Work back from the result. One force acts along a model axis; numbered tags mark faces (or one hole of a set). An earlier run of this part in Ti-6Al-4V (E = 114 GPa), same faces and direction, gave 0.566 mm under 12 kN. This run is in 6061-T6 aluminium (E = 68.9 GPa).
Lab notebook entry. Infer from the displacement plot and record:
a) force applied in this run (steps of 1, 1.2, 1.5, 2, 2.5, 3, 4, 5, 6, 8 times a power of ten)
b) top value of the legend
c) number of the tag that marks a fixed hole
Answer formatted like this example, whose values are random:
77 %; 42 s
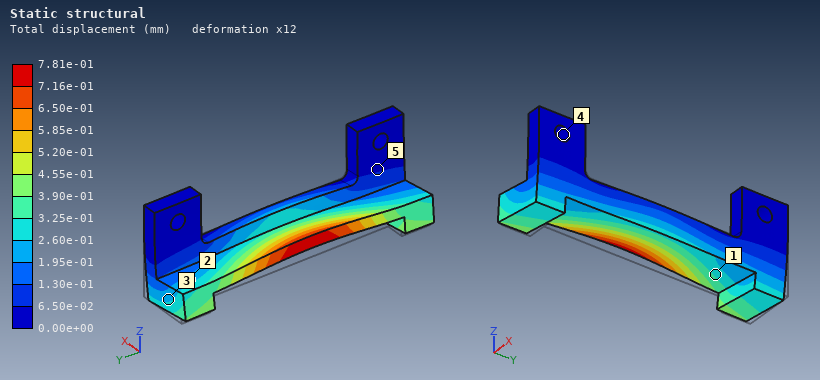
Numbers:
10 kN; 7.81e-01 mm; 4
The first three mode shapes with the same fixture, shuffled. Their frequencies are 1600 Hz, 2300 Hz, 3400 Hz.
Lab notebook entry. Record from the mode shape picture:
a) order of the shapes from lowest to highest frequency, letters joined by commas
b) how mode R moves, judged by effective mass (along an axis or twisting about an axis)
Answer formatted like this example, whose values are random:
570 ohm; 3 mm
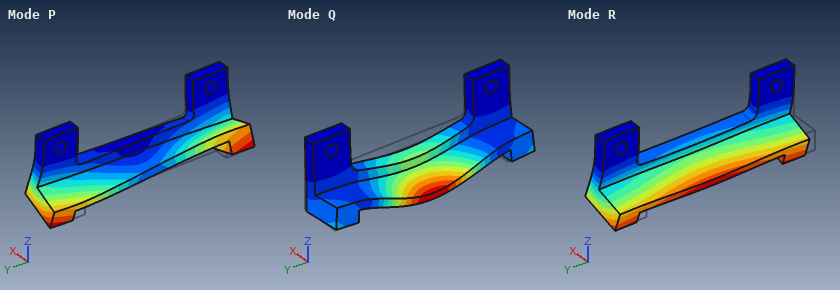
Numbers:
R, P, Q; along X
